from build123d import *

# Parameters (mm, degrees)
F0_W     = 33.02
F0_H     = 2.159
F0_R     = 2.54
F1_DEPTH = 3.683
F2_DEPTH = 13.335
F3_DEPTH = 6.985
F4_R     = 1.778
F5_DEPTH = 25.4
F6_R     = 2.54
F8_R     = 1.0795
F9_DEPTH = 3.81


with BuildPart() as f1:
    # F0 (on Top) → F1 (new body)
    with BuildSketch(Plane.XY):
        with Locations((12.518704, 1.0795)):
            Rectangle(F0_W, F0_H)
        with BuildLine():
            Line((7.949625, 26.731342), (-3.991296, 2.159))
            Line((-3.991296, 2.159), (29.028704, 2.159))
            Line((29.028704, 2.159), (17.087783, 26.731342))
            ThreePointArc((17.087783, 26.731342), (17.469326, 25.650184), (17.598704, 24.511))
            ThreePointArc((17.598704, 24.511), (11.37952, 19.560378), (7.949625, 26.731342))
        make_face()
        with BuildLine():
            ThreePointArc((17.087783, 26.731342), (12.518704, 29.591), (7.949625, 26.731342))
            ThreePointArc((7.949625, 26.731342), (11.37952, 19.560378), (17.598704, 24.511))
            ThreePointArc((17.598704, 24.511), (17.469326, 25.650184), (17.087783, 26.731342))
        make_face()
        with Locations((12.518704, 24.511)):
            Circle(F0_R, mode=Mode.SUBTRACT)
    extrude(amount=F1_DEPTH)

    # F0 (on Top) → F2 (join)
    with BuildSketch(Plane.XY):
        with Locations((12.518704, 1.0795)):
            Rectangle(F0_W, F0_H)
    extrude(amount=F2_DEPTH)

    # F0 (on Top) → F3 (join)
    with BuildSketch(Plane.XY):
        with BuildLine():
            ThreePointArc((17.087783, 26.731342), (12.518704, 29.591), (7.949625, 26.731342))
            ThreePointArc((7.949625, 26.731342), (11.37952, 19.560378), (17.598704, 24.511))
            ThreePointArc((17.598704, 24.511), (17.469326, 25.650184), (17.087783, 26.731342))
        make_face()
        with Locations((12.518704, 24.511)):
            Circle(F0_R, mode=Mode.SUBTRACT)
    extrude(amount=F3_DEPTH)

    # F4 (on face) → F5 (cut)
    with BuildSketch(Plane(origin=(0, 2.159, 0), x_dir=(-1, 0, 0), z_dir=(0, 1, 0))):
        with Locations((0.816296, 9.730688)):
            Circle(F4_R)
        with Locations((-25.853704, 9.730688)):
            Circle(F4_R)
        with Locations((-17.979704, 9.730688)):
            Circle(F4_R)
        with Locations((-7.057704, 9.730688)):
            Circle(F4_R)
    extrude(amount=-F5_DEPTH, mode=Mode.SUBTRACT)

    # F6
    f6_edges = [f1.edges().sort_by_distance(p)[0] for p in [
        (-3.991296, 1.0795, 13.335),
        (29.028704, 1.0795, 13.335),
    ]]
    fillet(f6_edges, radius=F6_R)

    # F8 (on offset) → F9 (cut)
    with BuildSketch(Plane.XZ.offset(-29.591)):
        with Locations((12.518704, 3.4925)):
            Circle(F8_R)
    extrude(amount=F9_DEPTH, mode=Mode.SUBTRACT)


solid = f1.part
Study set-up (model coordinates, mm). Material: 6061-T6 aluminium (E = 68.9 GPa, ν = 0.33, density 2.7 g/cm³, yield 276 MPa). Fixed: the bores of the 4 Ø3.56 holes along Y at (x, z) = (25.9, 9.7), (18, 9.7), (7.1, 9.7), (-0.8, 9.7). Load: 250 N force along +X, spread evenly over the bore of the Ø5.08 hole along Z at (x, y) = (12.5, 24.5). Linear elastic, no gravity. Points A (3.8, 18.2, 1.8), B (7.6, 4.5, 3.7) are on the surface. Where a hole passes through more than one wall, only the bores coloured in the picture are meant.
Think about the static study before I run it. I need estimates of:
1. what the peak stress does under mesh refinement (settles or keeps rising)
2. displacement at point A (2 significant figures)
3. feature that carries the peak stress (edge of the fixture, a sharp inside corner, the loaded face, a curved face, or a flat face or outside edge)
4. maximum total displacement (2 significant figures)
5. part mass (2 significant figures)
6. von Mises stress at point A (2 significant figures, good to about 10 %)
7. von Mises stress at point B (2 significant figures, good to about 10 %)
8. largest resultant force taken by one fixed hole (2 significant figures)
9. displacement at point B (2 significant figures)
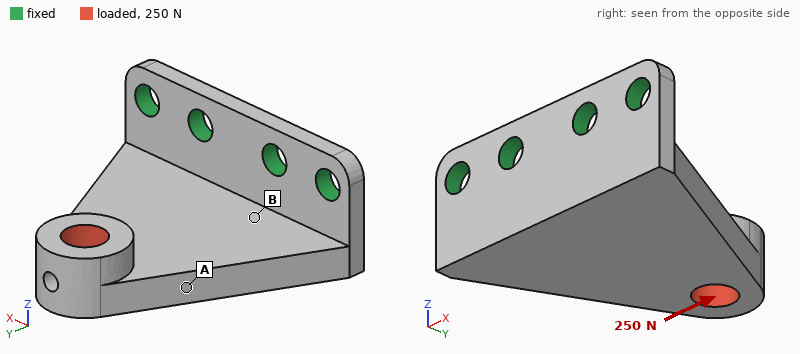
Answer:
keeps rising
33 µm
edge of the fixture
55 µm
8.0 g
12 MPa
28 MPa
200 N
8.5 µm
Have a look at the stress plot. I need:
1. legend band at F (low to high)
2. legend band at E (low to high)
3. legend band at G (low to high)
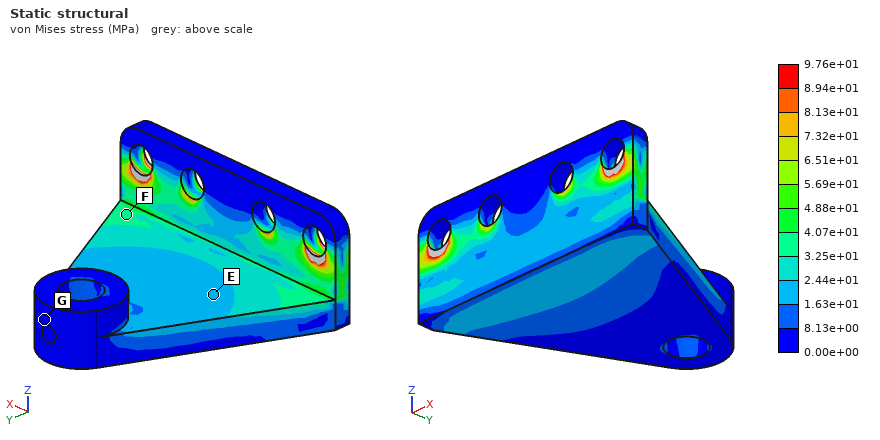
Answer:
3.25e+01 to 4.07e+01 MPa
1.63e+01 to 2.44e+01 MPa
0.00e+00 to 8.13e+00 MPa
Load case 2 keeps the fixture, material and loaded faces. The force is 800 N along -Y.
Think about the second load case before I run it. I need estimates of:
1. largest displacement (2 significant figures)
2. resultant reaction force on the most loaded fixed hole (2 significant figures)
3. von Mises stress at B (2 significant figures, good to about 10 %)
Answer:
83 µm
230 N
28 MPa
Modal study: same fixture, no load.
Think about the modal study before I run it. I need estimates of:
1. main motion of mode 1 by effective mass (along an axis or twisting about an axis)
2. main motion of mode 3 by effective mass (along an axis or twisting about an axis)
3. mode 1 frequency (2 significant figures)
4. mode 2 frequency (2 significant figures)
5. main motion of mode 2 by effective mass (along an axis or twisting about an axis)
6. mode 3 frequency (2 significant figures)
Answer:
along Z
along Y
2400 Hz
7900 Hz
along X
12 kHz
